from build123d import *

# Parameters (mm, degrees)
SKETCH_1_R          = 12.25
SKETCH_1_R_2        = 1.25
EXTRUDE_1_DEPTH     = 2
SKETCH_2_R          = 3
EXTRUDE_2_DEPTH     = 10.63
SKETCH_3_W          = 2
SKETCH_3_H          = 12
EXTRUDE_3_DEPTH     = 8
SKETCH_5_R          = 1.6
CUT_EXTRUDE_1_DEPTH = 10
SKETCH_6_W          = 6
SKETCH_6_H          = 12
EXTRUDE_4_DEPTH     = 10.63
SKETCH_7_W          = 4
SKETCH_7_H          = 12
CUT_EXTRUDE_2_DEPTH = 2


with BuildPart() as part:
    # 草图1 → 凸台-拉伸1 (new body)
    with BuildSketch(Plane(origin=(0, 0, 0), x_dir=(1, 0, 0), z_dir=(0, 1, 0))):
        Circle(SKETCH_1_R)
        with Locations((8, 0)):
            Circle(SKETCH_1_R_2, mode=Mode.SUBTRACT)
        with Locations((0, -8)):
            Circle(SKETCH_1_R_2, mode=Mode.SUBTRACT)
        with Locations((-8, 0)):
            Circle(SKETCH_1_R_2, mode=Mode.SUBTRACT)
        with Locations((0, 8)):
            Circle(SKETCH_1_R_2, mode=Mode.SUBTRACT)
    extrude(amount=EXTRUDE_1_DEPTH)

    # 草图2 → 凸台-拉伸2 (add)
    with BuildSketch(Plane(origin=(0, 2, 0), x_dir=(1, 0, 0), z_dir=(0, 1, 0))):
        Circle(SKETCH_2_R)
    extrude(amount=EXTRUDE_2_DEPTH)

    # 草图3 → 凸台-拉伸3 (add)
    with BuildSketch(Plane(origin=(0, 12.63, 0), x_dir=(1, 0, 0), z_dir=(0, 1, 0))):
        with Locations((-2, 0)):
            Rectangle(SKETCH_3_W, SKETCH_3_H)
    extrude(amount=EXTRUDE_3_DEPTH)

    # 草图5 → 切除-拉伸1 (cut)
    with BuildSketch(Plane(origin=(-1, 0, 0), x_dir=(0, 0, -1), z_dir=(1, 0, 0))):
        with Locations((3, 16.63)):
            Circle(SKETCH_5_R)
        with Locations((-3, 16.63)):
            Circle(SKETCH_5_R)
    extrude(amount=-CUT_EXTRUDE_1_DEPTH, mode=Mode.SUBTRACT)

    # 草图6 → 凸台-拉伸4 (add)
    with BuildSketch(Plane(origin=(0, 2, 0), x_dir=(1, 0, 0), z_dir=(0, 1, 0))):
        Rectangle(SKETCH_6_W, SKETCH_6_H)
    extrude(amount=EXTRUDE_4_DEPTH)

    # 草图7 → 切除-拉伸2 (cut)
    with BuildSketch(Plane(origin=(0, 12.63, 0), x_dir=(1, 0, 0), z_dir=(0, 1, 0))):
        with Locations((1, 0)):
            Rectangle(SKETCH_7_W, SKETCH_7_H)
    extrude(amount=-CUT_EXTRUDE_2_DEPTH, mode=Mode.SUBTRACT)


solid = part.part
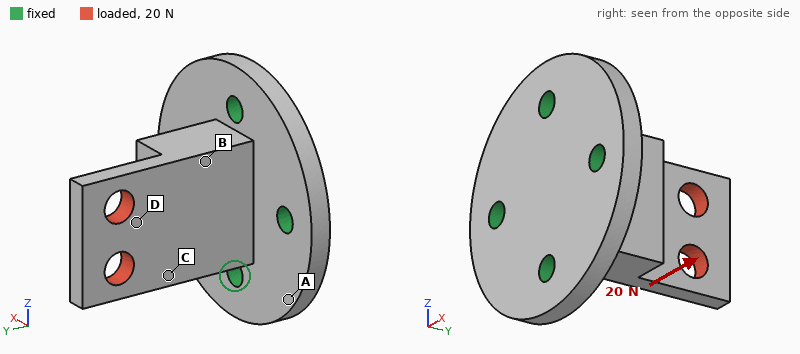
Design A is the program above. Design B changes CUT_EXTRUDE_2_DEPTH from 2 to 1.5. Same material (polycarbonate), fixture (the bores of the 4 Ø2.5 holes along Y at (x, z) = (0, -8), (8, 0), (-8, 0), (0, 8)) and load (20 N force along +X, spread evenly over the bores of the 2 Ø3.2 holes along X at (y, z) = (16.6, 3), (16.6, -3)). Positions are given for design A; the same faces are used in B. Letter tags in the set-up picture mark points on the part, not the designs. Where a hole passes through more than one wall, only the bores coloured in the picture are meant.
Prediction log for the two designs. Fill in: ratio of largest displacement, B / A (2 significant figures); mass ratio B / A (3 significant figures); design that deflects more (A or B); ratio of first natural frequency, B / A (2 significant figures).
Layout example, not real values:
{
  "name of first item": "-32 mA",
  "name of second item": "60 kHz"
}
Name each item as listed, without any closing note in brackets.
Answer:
{
  "ratio of largest displacement, B / A": "0.91",
  "mass ratio B / A": "1.01",
  "design that deflects more": "A",
  "ratio of first natural frequency, B / A": "1.0"
}
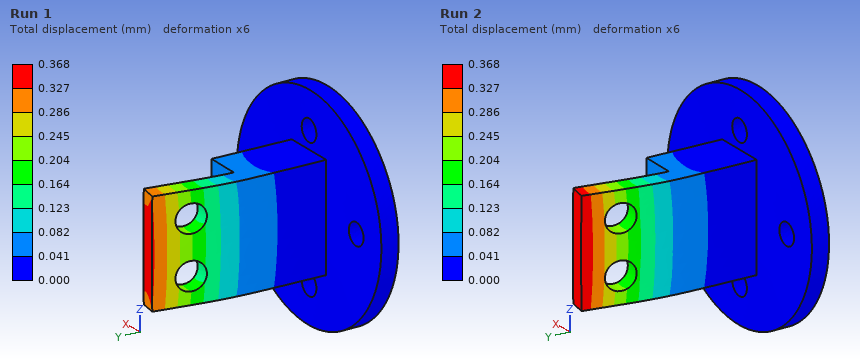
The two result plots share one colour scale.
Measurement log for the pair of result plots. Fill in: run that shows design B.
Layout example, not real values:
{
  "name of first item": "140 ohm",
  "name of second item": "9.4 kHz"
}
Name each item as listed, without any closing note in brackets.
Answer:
{
  "run that shows design B": "Run 1"
}
